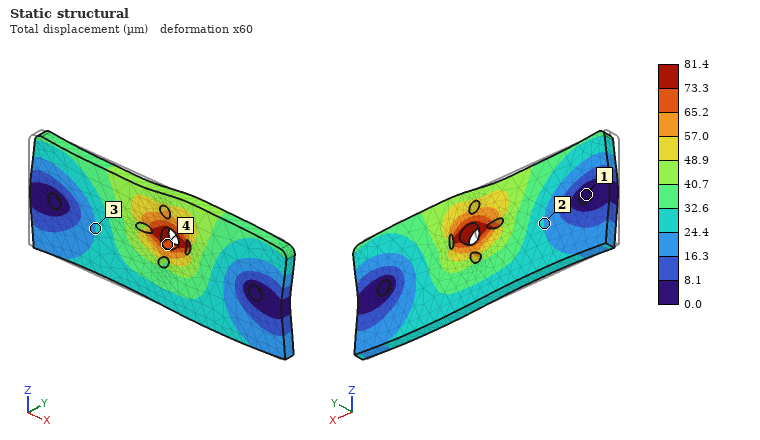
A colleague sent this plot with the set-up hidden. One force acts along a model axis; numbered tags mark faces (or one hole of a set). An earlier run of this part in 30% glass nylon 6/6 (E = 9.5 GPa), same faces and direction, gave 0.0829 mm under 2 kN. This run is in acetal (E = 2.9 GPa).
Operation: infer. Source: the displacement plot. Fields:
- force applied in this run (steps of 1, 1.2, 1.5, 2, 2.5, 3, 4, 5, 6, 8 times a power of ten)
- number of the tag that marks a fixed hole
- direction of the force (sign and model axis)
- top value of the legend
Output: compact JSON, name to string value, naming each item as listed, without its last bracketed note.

{"force applied in this run": "600 N", "number of the tag that marks a fixed hole": "1", "direction of the force": "+X", "top value of the legend": "81.4 µm"}
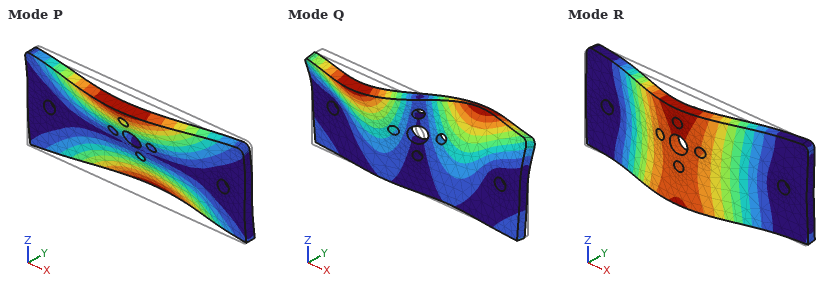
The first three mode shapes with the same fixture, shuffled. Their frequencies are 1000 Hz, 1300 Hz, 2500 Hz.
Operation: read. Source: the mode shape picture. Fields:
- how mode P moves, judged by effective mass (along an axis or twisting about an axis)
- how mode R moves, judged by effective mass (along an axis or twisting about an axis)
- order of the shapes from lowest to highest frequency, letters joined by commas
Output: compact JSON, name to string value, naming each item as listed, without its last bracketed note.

{"how mode P moves, judged by effective mass": "twisting about X", "how mode R moves, judged by effective mass": "along Y", "order of the shapes from lowest to highest frequency, letters joined by commas": "R, P, Q"}
